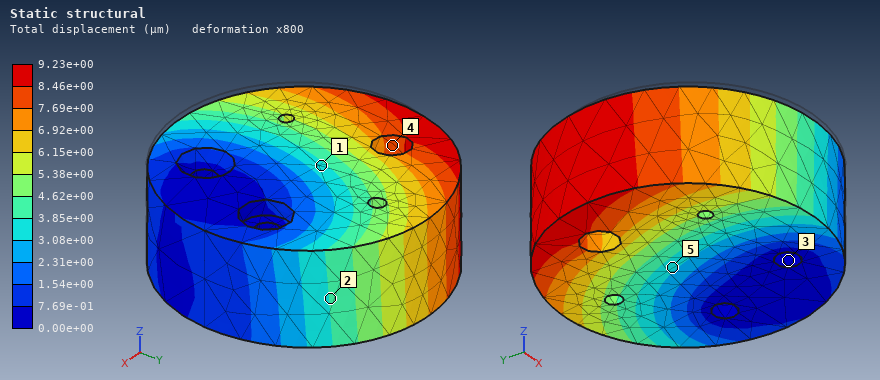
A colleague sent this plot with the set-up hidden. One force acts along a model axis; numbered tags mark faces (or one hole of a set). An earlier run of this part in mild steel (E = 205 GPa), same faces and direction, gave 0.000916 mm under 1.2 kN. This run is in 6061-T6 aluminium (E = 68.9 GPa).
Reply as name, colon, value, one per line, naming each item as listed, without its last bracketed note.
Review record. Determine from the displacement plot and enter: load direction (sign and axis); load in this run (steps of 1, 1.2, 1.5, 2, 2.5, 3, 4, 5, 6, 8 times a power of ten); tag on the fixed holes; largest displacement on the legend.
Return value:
load direction: +Y
load in this run: 4 kN
tag on the fixed holes: 3
largest displacement on the legend: 9.23e+00 µm
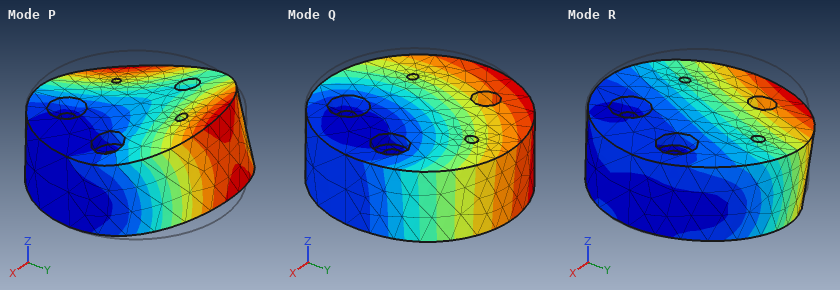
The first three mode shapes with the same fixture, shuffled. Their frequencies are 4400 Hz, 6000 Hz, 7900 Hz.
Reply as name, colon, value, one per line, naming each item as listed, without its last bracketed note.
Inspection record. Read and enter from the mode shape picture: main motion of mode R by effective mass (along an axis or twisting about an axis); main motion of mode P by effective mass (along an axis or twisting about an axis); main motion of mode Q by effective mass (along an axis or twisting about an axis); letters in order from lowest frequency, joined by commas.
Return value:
main motion of mode R by effective mass: along Z
main motion of mode P by effective mass: twisting about X
main motion of mode Q by effective mass: along Y
letters in order from lowest frequency, joined by commas: R, Q, P
